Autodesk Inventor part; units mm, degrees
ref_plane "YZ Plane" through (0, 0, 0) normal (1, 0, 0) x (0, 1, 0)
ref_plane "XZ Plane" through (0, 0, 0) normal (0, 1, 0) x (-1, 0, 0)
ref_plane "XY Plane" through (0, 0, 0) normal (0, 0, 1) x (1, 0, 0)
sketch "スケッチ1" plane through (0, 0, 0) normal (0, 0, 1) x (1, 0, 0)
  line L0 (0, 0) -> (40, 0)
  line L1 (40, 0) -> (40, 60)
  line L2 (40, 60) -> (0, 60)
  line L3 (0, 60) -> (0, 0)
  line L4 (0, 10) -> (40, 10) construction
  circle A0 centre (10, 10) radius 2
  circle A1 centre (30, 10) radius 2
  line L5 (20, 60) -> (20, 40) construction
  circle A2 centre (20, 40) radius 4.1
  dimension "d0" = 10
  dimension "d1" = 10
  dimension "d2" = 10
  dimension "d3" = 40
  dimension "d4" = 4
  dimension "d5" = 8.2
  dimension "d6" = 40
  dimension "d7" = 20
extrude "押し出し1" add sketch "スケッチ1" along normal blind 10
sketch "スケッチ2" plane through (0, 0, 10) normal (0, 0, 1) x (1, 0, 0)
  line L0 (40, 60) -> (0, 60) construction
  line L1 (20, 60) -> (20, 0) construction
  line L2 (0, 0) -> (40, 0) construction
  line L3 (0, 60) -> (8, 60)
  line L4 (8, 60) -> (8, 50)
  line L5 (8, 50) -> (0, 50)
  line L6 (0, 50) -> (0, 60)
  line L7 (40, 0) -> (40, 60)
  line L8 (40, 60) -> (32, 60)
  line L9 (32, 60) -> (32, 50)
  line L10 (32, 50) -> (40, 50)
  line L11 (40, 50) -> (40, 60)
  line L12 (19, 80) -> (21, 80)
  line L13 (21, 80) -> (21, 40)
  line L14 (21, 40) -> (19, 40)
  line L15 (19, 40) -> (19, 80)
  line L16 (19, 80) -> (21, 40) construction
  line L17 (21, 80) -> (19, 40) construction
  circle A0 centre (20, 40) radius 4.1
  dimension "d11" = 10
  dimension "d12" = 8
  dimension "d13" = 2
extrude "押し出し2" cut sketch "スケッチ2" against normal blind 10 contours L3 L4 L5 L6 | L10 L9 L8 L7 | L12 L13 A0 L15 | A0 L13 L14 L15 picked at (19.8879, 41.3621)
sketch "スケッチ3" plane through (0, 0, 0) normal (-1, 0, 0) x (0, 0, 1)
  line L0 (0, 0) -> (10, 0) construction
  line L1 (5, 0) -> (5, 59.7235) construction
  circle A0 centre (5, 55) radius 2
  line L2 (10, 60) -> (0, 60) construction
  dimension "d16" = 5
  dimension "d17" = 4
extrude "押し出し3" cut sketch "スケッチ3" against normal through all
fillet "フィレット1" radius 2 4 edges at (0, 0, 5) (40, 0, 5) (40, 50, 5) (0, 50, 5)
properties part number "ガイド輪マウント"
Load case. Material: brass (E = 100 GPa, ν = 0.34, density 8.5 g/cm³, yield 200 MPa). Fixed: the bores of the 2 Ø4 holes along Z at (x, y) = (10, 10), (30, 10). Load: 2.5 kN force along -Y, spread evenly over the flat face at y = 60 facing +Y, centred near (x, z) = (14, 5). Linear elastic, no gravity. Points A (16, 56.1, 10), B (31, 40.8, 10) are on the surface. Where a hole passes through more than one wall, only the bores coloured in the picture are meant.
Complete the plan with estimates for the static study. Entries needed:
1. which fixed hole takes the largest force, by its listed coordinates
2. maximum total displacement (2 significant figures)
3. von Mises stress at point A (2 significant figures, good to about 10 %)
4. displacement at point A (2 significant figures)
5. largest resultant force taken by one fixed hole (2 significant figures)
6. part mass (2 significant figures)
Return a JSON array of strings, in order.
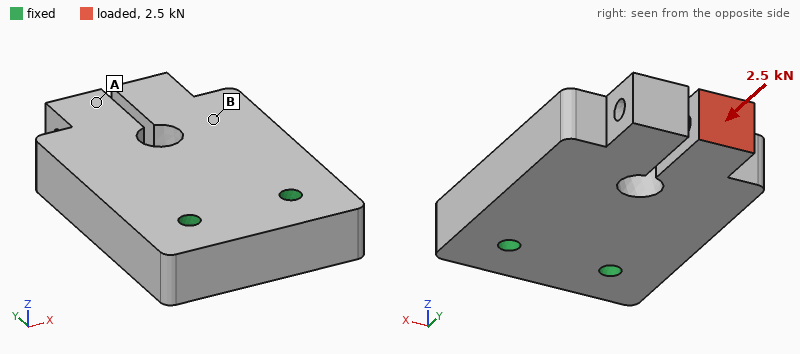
["(10, 10)", "19 µm", "18 MPa", "14 µm", "2.0 kN", "180 g"]
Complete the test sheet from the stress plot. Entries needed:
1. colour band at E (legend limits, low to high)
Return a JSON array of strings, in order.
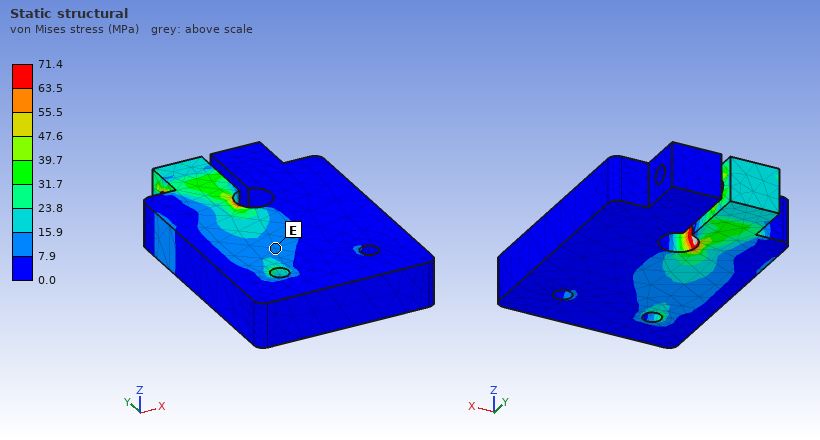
["7.9 to 15.9 MPa"]
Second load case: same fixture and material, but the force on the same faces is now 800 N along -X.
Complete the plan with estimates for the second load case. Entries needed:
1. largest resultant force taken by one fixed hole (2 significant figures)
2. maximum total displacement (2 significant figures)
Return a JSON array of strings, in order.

["1.9 kN", "47 µm"]
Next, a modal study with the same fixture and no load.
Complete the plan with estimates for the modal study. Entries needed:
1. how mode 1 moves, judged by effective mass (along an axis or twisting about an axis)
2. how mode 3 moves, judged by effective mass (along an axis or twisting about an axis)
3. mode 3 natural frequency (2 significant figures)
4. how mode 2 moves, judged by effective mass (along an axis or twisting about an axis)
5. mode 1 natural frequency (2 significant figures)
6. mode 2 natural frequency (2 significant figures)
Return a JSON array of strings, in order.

["along Z", "along X", "5800 Hz", "twisting about Y", "2500 Hz", "4400 Hz"]
